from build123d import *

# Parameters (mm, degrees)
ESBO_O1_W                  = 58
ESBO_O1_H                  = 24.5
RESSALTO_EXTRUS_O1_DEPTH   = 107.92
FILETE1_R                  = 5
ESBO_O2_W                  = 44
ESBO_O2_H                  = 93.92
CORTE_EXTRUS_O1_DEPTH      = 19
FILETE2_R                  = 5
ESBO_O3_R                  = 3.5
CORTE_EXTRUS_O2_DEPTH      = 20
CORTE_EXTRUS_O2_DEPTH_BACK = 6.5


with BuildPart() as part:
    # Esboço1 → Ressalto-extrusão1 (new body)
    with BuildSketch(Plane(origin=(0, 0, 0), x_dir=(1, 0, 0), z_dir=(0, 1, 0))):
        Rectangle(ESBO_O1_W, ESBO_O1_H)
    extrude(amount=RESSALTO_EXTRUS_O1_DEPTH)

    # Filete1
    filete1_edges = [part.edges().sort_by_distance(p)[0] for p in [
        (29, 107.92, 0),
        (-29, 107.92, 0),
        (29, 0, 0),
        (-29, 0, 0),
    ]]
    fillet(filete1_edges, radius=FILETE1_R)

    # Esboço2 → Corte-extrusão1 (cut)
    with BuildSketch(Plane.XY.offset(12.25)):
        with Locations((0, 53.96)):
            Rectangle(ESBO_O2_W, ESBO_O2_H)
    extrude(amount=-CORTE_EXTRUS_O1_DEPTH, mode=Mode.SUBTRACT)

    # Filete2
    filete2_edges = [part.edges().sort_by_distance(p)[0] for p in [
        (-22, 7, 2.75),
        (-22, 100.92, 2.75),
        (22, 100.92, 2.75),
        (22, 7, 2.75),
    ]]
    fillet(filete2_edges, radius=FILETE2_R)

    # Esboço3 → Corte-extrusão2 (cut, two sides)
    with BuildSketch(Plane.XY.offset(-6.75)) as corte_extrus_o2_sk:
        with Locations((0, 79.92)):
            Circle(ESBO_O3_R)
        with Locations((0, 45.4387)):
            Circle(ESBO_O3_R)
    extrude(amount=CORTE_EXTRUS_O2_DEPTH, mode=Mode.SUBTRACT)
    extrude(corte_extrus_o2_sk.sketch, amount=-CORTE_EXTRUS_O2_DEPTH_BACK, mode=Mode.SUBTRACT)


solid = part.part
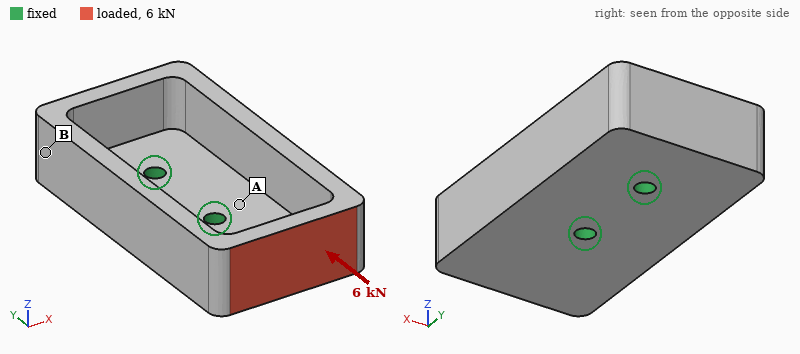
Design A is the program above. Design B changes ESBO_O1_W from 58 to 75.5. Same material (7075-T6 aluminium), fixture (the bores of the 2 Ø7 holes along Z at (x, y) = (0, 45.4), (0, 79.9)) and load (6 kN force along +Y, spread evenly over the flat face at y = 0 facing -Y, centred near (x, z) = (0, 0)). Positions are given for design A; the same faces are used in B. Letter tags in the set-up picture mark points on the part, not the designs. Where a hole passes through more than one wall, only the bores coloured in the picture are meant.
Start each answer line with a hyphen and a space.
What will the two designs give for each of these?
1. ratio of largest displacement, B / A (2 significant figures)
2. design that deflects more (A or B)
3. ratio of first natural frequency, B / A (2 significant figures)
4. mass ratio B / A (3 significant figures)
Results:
- 0.75
- A
- 0.65
- 1.62
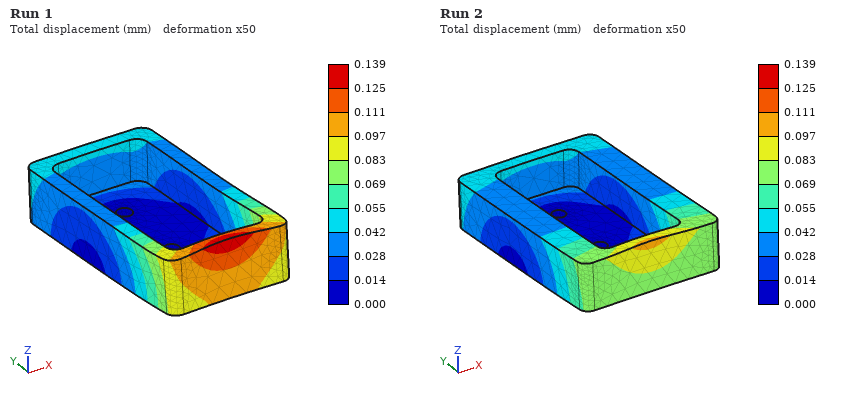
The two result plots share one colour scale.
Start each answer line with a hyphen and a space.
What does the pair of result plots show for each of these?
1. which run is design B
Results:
- Run 2
